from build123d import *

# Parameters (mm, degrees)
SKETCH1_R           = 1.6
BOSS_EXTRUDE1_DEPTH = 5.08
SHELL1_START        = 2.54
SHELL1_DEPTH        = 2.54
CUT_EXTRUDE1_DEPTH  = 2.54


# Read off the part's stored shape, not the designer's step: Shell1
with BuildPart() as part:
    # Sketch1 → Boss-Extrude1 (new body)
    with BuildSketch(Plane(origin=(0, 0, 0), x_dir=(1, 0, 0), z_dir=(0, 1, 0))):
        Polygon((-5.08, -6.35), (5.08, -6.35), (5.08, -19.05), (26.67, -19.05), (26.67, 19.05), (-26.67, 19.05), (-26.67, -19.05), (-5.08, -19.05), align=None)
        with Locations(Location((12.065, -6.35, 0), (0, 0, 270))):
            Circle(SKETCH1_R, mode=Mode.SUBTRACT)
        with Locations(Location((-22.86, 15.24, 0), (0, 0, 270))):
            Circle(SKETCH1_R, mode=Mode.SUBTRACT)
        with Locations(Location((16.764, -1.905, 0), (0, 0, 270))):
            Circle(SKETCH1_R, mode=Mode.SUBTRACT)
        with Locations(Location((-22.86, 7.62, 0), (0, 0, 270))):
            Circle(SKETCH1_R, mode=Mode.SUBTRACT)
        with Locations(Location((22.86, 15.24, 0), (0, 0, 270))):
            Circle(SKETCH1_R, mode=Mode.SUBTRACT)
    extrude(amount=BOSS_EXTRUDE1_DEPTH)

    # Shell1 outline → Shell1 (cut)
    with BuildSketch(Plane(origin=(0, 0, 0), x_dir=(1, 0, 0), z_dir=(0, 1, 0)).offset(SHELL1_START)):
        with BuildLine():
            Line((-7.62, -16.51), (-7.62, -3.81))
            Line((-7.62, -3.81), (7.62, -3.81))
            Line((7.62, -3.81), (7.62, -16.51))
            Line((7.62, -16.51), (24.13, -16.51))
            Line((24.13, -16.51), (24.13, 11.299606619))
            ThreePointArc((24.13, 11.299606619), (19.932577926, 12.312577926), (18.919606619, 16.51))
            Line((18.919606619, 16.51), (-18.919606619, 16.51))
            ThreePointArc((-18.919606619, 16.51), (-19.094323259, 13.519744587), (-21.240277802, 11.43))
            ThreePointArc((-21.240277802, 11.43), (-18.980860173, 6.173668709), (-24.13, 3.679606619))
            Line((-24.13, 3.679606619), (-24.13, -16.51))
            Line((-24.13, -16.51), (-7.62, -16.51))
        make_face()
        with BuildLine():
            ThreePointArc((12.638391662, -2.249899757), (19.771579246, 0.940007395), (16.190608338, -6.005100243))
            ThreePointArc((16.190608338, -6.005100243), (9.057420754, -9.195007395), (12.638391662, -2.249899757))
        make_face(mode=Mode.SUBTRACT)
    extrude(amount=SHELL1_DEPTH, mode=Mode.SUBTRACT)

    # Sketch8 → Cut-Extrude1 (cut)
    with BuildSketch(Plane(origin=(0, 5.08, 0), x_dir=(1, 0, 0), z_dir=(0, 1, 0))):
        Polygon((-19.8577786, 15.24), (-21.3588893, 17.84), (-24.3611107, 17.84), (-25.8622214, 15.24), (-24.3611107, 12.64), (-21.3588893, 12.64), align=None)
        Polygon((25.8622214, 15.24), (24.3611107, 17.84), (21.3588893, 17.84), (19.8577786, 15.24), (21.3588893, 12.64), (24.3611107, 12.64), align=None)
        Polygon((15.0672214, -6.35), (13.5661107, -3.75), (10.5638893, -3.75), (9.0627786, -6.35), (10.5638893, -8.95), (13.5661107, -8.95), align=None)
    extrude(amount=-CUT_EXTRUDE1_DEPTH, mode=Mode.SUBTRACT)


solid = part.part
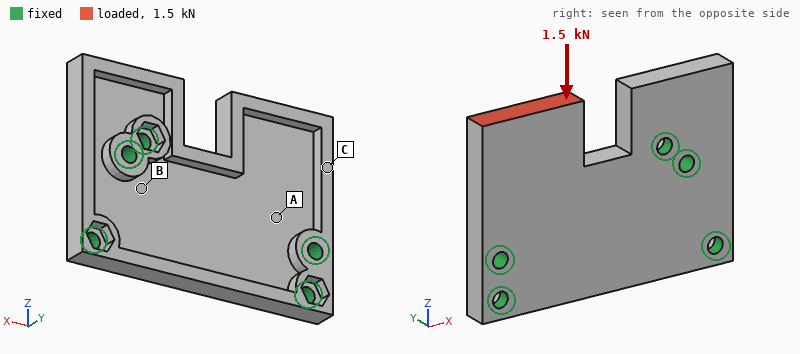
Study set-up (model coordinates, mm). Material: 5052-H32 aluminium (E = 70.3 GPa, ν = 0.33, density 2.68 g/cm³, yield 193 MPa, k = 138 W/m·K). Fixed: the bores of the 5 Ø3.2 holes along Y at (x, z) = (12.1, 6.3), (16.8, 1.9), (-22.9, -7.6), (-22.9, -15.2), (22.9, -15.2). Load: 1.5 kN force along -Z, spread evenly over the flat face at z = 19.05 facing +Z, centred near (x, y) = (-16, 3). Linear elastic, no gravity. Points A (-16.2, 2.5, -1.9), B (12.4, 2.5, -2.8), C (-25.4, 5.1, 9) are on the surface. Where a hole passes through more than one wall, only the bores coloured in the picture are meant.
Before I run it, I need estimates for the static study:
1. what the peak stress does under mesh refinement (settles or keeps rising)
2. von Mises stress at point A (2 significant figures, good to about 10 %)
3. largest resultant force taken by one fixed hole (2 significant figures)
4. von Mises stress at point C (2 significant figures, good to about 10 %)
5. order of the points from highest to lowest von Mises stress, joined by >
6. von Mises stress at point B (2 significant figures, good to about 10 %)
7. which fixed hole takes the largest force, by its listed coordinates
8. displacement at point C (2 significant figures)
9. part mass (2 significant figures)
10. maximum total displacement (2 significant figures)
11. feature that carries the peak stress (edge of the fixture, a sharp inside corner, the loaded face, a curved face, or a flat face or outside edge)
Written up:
keeps rising
38 MPa
990 N
66 MPa
C > A > B
9.7 MPa
(-22.9, -7.6)
27 µm
17 g
87 µm
a sharp inside corner
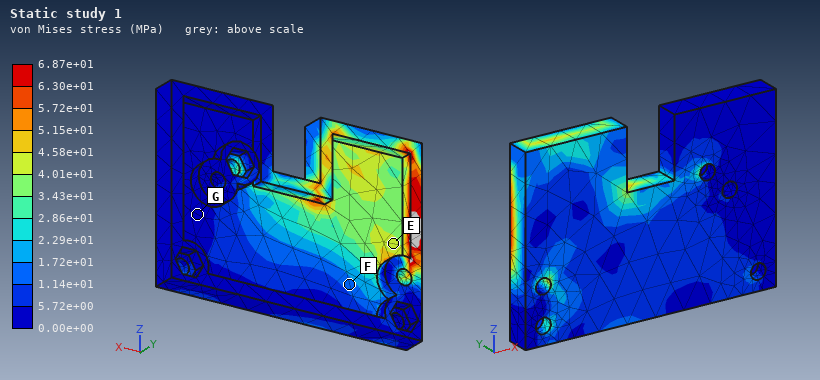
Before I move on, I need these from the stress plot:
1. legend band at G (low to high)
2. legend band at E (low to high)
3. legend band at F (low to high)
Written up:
0.00e+00 to 5.72e+00 MPa
4.01e+01 to 4.58e+01 MPa
1.14e+01 to 1.72e+01 MPa
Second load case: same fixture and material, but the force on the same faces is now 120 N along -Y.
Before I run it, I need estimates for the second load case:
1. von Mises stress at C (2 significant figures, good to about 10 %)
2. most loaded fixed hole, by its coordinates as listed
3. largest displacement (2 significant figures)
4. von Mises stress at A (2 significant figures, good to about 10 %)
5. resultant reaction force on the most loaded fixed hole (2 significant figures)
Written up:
41 MPa
(-22.9, -7.6)
0.12 mm
27 MPa
130 N
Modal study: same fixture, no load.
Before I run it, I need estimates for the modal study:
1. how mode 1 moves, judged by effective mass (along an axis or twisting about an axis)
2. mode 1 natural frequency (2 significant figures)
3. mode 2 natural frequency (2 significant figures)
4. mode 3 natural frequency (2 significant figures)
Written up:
along Y
4300 Hz
9700 Hz
11 kHz
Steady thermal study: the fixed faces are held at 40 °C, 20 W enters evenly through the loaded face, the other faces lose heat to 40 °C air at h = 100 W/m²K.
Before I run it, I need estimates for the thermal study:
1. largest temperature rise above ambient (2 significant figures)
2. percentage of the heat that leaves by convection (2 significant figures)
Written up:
49 K
22 %
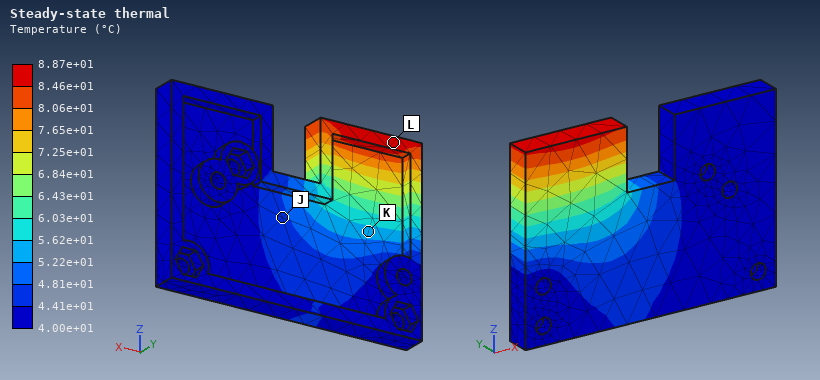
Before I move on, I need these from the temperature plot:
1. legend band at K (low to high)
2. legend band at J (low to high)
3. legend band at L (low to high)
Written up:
5.22e+01 to 5.62e+01 °C
4.41e+01 to 4.81e+01 °C
8.46e+01 to 8.87e+01 °C
